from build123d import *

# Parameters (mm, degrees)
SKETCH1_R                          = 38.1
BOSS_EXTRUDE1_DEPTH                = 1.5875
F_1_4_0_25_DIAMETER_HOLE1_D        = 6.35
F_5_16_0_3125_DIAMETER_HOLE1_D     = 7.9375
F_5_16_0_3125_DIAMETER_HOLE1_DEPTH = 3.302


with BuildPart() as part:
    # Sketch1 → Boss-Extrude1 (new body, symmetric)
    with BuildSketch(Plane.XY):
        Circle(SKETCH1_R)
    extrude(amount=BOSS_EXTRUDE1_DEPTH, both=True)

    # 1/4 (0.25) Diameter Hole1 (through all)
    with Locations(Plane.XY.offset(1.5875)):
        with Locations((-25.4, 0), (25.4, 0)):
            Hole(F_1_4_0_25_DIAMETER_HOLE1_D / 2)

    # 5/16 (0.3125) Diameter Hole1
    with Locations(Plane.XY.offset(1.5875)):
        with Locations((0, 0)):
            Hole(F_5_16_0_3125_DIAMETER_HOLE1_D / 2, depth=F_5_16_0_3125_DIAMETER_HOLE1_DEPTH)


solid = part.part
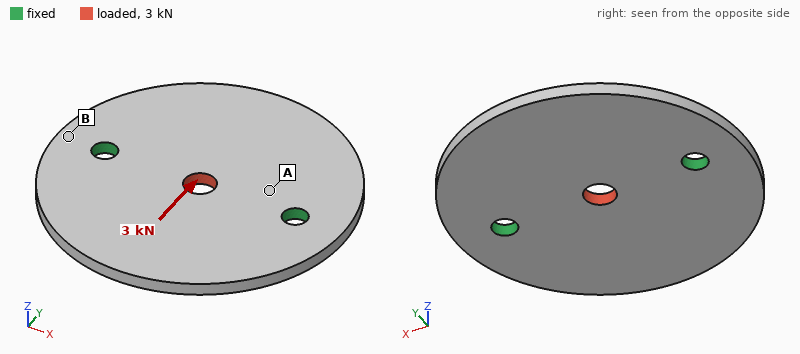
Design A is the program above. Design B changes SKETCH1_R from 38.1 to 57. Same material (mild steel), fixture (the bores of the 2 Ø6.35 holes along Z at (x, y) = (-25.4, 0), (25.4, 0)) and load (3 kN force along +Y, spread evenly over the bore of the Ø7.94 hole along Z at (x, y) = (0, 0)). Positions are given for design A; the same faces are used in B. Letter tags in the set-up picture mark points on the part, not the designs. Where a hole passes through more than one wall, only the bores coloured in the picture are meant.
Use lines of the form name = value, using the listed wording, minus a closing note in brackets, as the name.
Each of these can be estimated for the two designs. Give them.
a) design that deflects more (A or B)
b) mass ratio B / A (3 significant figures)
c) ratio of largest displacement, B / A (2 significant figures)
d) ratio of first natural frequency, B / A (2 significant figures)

design that deflects more = A
mass ratio B / A = 2.27
ratio of largest displacement, B / A = 0.90
ratio of first natural frequency, B / A = 0.46
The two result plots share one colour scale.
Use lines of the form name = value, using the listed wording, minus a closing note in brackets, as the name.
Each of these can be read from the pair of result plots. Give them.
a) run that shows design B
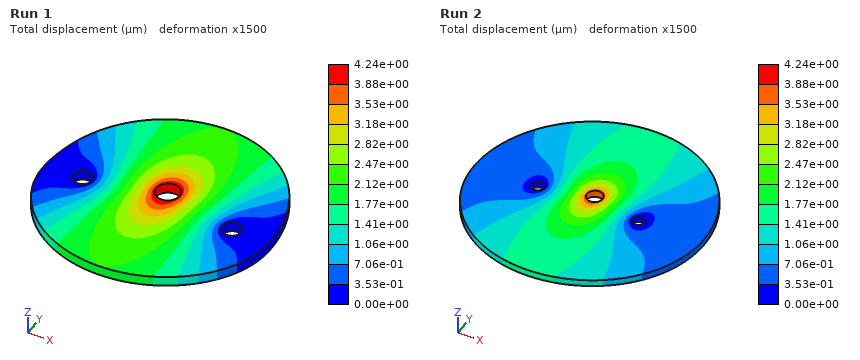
run that shows design B = Run 2
